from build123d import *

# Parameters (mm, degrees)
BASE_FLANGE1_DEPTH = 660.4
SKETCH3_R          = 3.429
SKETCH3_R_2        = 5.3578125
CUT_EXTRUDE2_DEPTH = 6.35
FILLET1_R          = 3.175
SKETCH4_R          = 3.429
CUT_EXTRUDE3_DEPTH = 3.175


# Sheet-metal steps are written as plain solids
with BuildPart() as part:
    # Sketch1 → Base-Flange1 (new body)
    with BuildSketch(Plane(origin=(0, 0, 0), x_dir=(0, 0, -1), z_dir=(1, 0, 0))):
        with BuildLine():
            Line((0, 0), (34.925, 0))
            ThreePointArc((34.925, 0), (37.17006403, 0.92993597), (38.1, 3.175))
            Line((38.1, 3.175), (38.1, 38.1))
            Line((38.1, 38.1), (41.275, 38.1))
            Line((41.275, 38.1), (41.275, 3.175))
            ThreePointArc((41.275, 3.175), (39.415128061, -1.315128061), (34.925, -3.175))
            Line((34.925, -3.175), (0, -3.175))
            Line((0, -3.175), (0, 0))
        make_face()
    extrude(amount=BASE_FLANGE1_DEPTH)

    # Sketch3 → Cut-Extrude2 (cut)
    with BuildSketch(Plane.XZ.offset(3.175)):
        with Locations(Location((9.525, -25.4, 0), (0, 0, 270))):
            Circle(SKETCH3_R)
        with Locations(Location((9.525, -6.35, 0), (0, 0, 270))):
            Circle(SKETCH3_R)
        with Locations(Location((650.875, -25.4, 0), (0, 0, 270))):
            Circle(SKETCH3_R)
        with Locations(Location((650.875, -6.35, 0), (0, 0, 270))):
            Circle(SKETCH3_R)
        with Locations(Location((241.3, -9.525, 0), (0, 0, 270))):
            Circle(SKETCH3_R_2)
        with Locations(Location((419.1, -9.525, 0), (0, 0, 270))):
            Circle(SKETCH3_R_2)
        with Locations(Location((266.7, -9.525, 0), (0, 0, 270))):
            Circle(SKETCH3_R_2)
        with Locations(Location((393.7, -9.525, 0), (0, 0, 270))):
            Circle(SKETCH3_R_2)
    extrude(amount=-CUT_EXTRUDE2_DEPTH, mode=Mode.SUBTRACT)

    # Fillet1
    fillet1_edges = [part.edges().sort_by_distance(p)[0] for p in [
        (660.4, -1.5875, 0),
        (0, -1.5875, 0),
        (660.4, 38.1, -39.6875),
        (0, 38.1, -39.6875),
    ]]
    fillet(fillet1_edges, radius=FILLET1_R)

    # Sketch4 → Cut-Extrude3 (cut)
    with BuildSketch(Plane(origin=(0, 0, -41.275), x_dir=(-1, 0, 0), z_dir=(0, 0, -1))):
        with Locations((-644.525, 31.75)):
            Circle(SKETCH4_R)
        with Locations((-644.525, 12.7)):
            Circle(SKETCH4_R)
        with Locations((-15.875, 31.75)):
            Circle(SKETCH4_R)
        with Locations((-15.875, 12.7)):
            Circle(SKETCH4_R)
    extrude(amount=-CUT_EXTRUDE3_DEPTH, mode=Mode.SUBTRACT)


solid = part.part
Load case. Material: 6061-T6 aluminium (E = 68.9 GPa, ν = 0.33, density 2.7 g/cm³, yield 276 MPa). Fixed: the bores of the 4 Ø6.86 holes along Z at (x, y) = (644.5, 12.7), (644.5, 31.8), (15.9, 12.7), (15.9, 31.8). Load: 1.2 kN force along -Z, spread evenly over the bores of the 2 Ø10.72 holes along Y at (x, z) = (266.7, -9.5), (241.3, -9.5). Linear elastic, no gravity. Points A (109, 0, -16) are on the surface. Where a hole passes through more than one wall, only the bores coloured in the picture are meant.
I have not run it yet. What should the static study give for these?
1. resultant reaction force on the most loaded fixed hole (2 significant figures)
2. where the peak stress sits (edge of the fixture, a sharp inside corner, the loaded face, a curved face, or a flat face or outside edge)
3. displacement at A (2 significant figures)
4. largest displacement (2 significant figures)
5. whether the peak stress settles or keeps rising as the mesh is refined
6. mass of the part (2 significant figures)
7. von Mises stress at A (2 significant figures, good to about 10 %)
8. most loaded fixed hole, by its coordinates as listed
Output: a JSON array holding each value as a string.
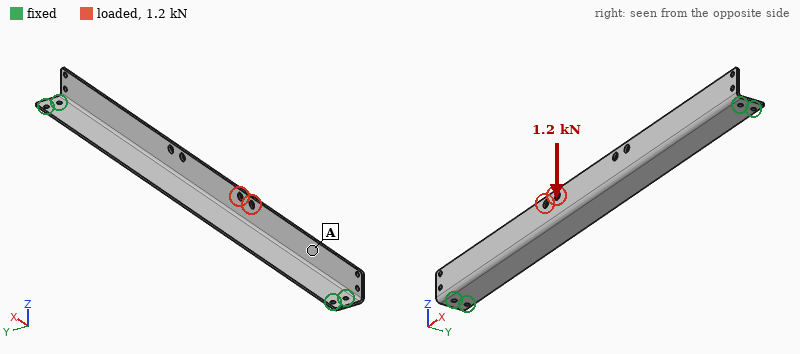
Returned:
["4.9 kN", "edge of the fixture", "1.0 mm", "2.4 mm", "keeps rising", "430 g", "25 MPa", "(15.9, 12.7)"]
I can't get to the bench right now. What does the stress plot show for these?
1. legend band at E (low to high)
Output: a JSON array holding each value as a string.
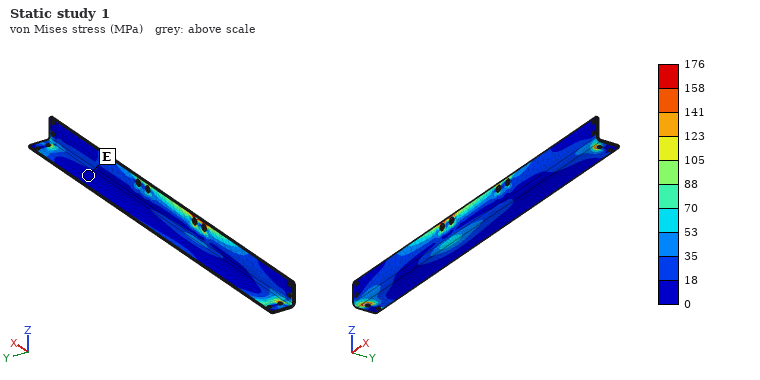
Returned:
["0 to 18 MPa"]
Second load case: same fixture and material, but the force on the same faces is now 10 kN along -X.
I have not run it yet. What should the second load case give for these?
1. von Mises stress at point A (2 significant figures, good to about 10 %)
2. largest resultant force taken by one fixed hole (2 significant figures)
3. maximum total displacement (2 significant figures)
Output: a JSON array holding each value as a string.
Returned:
["21 MPa", "4.1 kN", "0.87 mm"]
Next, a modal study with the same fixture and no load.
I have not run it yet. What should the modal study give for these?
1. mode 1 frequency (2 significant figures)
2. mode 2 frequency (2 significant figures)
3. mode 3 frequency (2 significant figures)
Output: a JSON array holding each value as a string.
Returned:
["190 Hz", "260 Hz", "400 Hz"]
